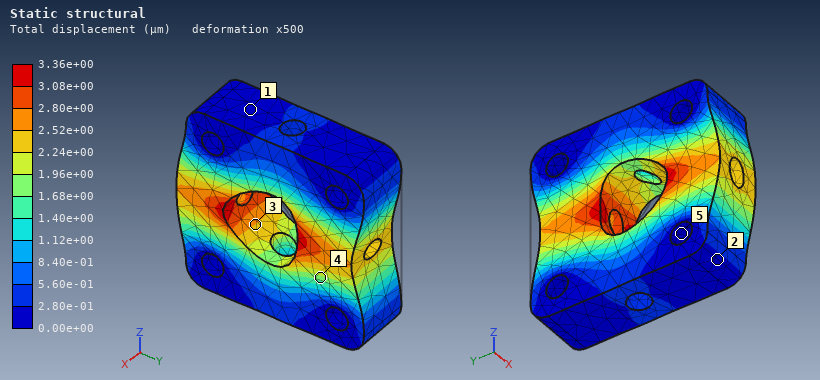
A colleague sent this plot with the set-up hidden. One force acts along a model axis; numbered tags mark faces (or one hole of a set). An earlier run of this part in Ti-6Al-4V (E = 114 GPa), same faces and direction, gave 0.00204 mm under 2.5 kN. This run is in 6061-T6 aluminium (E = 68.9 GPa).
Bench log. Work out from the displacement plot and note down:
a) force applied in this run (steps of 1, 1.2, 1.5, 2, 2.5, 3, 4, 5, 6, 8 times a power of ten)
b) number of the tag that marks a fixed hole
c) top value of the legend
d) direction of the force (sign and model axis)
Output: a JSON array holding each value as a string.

["2.5 kN", "5", "3.36e+00 µm", "-Y"]
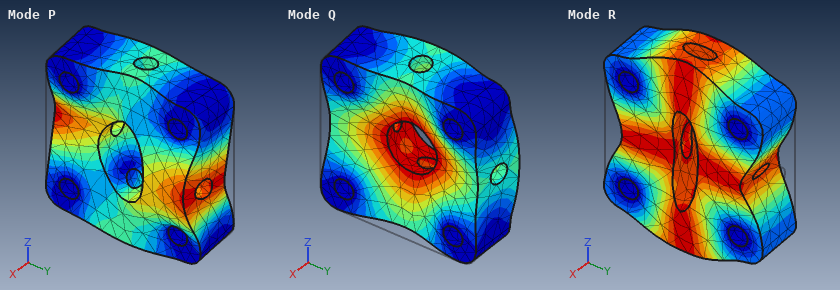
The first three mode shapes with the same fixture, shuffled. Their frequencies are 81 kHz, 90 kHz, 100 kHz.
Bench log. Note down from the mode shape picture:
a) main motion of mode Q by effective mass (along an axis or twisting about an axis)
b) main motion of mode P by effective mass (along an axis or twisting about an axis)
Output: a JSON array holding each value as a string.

["along X", "twisting about Z"]
